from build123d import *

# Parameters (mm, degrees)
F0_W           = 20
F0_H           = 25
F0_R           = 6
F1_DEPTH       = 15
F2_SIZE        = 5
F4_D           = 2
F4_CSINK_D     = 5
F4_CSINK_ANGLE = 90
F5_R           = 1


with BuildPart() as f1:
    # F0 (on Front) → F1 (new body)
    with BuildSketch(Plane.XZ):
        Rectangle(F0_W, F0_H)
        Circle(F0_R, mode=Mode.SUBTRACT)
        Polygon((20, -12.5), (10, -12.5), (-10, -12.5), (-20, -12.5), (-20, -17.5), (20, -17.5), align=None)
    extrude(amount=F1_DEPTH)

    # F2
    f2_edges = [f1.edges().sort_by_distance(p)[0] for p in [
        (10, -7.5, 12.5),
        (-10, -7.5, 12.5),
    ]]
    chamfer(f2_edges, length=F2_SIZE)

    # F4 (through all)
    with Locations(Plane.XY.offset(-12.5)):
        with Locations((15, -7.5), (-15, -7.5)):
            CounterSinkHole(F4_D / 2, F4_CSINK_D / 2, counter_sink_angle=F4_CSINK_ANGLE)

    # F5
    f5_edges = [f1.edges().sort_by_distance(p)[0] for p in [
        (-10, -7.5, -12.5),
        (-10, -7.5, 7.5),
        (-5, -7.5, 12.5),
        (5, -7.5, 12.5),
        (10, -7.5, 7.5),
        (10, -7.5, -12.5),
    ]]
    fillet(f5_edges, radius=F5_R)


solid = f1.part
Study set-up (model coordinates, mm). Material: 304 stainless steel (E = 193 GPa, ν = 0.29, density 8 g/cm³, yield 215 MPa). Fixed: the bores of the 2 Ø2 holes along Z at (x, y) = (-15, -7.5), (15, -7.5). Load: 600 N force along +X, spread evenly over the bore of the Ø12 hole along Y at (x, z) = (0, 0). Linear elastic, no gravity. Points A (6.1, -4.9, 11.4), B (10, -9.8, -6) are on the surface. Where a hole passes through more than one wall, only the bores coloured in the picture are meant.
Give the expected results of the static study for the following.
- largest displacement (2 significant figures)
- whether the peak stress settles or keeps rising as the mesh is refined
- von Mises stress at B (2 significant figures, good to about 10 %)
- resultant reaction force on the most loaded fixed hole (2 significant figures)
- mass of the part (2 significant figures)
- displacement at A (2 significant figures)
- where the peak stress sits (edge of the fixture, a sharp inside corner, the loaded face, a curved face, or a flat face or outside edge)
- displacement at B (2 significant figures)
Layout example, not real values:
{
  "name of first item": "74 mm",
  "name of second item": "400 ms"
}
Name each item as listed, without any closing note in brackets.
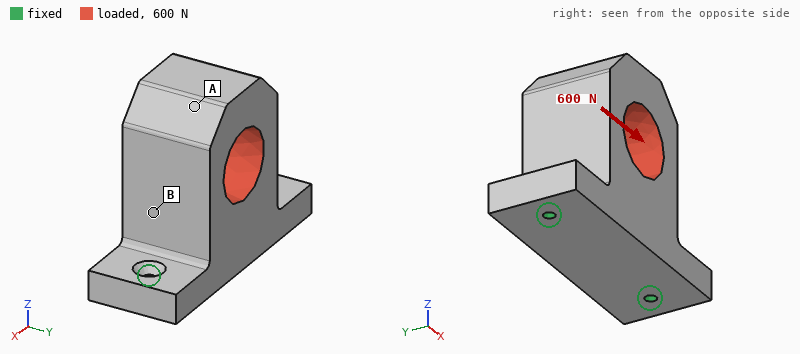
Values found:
{
  "largest displacement": "4.9 µm",
  "whether the peak stress settles or keeps rising as the mesh is refined": "keeps rising",
  "von Mises stress at B": "10 MPa",
  "resultant reaction force on the most loaded fixed hole": "450 N",
  "mass of the part": "67 g",
  "displacement at A": "4.8 µm",
  "where the peak stress sits": "edge of the fixture",
  "displacement at B": "1.9 µm"
}
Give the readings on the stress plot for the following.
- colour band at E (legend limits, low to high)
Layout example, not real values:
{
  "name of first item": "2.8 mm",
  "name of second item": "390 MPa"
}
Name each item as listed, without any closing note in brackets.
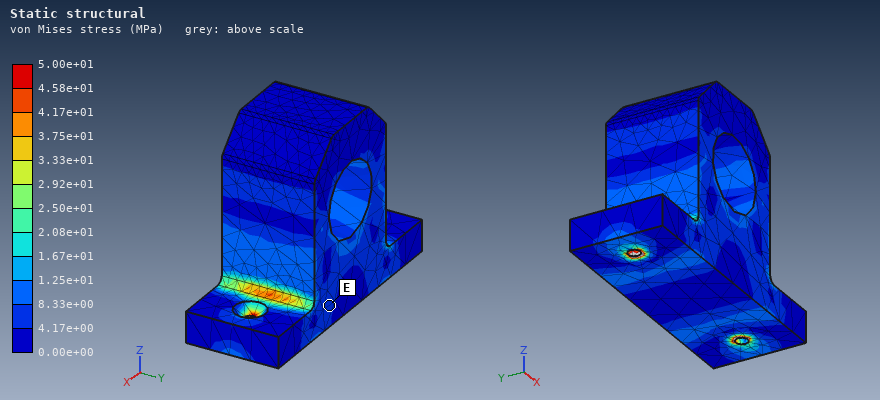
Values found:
{
  "colour band at E": "4.17e+00 to 8.33e+00 MPa"
}
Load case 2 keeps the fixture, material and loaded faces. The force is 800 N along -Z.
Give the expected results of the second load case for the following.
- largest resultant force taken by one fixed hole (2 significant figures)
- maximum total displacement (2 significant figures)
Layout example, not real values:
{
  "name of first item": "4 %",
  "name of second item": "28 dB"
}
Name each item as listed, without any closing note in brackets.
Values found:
{
  "largest resultant force taken by one fixed hole": "460 N",
  "maximum total displacement": "2.2 µm"
}
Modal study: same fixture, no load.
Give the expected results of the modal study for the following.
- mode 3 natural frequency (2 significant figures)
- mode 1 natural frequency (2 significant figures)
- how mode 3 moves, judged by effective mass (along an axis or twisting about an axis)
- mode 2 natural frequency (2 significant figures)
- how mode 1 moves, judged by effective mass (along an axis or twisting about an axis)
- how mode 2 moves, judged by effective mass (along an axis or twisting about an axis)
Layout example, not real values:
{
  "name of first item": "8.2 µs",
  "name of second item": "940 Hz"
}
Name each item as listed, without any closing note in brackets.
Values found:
{
  "mode 3 natural frequency": "14 kHz",
  "mode 1 natural frequency": "3400 Hz",
  "how mode 3 moves, judged by effective mass": "along Z",
  "mode 2 natural frequency": "9800 Hz",
  "how mode 1 moves, judged by effective mass": "along Y",
  "how mode 2 moves, judged by effective mass": "along X"
}
